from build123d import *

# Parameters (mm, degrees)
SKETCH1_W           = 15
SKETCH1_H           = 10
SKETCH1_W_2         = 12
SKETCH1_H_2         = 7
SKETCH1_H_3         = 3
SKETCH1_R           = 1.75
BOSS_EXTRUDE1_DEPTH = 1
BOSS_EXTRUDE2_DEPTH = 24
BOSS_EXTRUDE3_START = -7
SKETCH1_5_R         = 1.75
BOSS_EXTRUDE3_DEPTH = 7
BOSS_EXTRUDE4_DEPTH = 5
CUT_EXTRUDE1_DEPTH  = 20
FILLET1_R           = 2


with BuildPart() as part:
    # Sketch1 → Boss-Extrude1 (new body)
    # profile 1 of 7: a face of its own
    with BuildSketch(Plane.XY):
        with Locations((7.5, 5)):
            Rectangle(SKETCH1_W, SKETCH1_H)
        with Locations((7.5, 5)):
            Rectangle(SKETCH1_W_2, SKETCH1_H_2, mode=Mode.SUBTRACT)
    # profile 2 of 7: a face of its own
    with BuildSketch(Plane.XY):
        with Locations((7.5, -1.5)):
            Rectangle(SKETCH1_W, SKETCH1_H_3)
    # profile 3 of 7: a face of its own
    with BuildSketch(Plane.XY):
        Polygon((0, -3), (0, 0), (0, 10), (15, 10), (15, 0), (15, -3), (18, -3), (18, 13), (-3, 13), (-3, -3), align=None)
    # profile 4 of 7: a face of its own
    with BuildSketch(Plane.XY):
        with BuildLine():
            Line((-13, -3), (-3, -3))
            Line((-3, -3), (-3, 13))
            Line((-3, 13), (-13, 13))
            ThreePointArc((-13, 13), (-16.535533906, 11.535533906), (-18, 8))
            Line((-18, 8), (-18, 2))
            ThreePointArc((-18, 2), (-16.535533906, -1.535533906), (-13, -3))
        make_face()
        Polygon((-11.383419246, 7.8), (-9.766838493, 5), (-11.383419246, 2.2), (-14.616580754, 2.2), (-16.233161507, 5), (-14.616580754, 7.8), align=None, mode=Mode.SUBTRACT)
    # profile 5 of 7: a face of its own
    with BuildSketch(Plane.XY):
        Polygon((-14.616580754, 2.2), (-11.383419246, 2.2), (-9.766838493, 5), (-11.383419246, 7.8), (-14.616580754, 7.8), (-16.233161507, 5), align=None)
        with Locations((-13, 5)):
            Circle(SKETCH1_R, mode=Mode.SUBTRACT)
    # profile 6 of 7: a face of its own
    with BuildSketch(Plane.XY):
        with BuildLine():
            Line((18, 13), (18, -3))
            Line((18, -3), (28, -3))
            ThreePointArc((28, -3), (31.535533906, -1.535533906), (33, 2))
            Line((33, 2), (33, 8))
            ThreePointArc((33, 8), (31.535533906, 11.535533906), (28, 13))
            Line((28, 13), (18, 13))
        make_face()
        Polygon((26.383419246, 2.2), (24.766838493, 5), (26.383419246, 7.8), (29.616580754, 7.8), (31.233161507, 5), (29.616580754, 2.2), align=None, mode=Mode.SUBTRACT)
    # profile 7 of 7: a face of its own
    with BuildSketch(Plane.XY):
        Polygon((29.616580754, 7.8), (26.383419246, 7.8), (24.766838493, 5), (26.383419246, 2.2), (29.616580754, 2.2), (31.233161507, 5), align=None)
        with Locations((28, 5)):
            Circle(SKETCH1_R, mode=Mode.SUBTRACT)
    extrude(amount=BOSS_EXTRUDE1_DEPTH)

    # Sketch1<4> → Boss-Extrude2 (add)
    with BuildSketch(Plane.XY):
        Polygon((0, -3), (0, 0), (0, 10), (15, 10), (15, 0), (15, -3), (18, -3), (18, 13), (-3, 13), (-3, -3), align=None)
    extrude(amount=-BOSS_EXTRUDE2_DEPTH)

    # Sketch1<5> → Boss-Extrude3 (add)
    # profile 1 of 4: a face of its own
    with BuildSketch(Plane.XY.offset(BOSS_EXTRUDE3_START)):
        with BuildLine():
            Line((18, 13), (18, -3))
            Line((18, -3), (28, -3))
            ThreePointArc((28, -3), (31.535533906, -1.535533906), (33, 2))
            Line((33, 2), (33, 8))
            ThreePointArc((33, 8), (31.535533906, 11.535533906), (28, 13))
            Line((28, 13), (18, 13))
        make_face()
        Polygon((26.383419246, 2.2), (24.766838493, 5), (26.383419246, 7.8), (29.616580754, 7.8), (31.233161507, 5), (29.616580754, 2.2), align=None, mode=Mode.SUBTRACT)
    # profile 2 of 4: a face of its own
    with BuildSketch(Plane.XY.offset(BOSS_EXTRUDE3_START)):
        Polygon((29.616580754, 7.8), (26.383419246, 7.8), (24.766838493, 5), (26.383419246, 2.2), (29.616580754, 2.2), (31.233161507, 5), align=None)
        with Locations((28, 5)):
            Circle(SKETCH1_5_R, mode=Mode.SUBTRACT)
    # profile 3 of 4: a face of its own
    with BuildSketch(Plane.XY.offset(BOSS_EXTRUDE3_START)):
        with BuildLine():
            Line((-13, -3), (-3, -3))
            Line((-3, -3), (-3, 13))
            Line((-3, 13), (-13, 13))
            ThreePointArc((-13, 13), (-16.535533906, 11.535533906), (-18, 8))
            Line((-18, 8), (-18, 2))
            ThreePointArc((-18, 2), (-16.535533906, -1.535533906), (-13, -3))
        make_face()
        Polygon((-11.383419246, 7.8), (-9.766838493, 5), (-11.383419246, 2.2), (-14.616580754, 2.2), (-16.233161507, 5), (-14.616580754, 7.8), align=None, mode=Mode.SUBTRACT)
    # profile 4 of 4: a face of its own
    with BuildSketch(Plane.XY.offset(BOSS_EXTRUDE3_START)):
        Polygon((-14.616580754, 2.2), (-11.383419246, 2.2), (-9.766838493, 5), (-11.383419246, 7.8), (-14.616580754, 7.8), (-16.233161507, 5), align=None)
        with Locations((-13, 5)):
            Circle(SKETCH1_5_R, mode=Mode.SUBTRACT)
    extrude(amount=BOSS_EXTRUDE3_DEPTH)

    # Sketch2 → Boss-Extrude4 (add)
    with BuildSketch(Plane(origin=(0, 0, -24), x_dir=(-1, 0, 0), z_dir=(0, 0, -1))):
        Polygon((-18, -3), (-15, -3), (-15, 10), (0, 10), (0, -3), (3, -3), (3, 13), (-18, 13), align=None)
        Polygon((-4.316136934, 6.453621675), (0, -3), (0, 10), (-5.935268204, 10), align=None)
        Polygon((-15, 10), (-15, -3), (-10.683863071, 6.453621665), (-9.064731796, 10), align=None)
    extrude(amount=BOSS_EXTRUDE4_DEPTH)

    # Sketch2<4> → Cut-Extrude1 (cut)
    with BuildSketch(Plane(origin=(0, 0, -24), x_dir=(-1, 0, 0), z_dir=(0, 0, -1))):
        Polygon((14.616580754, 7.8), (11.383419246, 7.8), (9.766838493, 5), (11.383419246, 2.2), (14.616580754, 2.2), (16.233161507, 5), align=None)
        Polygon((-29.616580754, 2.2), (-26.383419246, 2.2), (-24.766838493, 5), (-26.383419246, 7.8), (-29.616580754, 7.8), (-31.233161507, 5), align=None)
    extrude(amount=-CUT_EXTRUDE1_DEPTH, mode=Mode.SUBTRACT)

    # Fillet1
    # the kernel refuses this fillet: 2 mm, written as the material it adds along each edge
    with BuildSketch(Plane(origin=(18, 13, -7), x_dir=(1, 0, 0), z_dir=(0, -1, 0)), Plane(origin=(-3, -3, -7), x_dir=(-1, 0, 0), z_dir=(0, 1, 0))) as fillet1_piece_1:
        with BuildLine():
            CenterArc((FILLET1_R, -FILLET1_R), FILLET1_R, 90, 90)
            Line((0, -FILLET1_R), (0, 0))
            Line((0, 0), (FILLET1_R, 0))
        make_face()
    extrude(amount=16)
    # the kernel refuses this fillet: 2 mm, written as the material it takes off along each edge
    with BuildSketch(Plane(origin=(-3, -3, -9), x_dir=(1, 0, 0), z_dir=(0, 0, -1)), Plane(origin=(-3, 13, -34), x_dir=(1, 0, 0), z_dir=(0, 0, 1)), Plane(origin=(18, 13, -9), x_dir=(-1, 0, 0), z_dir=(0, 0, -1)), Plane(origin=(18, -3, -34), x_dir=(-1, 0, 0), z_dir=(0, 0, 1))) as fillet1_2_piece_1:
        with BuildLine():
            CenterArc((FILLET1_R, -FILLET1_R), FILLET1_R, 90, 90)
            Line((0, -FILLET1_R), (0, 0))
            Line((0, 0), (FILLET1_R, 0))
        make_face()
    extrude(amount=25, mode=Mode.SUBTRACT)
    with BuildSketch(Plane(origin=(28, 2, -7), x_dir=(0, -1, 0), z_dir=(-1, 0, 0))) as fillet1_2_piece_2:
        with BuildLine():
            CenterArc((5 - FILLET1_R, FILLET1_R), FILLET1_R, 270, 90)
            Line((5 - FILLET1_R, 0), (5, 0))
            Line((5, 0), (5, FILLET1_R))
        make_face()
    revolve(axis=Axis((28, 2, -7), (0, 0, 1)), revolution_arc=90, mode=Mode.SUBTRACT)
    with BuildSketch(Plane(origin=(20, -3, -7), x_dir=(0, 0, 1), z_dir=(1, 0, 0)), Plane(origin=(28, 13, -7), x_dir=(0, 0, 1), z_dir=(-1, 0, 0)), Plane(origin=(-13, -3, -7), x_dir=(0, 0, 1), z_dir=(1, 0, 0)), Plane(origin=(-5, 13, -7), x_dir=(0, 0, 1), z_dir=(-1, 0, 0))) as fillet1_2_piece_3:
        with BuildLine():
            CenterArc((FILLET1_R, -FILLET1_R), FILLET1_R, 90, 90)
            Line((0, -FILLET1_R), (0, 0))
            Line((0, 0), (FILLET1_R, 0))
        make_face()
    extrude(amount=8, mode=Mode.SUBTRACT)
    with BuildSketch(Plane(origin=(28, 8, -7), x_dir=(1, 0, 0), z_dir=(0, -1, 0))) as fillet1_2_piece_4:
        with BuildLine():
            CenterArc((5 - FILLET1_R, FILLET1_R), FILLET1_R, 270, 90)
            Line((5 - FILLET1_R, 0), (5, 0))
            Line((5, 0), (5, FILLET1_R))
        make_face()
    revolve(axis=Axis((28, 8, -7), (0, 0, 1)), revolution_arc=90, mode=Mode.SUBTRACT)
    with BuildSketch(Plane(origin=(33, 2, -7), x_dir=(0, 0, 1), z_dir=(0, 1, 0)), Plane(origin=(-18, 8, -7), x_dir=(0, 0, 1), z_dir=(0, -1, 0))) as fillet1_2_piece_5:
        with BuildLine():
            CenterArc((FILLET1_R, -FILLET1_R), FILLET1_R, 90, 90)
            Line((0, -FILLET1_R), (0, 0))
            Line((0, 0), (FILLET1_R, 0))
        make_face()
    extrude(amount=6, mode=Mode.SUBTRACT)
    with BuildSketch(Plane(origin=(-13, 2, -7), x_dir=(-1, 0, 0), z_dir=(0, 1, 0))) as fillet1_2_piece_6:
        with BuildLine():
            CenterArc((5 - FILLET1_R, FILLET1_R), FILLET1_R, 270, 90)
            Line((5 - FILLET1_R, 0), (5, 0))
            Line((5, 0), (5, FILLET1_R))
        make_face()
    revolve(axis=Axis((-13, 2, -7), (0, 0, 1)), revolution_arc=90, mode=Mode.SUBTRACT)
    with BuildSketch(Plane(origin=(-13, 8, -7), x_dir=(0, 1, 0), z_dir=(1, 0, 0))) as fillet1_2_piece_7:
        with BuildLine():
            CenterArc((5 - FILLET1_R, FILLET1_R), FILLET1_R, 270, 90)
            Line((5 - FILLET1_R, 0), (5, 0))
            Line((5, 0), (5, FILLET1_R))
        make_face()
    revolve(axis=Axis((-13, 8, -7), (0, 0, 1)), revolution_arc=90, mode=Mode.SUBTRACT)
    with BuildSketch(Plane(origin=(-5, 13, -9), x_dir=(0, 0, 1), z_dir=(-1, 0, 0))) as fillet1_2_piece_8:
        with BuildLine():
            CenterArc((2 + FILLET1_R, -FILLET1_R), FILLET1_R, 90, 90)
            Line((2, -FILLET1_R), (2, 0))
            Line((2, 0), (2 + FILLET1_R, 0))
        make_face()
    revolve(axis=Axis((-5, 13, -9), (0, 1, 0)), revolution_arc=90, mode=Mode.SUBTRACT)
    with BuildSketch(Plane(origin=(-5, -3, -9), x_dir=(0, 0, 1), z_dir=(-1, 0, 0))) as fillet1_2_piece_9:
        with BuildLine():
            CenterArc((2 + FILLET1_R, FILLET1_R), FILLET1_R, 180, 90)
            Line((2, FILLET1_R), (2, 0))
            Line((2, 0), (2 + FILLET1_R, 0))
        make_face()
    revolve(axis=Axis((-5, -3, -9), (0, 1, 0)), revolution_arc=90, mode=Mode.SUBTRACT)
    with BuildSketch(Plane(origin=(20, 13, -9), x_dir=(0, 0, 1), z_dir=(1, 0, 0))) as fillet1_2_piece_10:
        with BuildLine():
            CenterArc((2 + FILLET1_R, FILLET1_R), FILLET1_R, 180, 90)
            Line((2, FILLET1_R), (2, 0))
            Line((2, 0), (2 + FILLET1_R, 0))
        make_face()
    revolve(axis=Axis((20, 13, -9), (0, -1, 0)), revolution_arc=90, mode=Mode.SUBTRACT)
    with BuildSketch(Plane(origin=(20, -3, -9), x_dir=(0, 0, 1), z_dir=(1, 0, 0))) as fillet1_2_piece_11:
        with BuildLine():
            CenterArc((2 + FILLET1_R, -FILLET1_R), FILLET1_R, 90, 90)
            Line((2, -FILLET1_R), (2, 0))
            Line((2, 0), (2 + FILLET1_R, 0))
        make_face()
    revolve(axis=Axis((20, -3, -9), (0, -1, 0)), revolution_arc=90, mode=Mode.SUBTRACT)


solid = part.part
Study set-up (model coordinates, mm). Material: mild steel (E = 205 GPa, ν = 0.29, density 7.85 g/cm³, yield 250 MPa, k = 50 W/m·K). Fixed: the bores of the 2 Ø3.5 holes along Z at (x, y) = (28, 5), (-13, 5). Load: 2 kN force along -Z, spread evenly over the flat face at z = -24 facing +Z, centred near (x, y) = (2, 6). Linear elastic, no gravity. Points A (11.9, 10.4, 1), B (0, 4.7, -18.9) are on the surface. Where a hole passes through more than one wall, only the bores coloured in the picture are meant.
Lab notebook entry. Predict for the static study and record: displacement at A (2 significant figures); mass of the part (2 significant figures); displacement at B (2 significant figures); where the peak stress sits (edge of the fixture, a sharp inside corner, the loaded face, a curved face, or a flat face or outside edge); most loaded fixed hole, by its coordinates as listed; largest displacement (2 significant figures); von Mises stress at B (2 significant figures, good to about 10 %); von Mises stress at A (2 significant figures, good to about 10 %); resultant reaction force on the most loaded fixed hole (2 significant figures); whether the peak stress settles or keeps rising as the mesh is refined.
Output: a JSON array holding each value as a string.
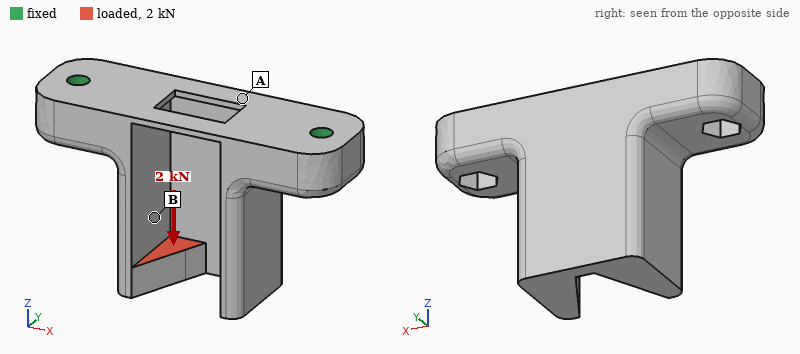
["6.4 µm", "63 g", "12 µm", "edge of the fixture", "(-13, 5)", "24 µm", "52 MPa", "20 MPa", "1.4 kN", "keeps rising"]
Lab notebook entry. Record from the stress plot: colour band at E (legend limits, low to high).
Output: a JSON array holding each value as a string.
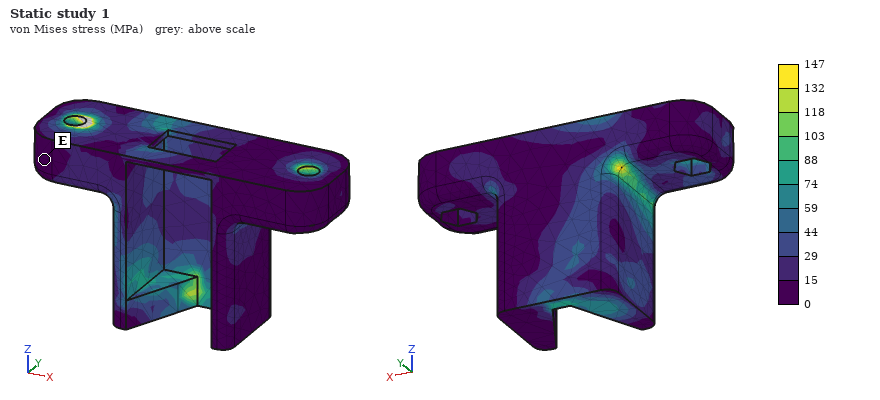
["0 to 15 MPa"]
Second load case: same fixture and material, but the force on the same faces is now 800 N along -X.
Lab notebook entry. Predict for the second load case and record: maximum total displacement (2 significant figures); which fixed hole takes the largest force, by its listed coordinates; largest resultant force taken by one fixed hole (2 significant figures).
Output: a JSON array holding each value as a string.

["44 µm", "(-13, 5)", "670 N"]
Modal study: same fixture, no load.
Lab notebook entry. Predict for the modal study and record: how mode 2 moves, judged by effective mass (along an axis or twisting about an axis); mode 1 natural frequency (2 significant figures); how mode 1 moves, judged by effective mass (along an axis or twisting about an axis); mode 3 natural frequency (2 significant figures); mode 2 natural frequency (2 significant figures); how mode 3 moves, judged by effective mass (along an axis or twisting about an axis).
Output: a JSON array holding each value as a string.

["along X", "5700 Hz", "along Y", "12 kHz", "7500 Hz", "along Z"]
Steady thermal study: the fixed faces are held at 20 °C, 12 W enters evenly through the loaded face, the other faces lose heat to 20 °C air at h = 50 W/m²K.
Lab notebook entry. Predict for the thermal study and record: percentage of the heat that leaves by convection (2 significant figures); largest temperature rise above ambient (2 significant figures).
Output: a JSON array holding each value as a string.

["32 %", "69 K"]
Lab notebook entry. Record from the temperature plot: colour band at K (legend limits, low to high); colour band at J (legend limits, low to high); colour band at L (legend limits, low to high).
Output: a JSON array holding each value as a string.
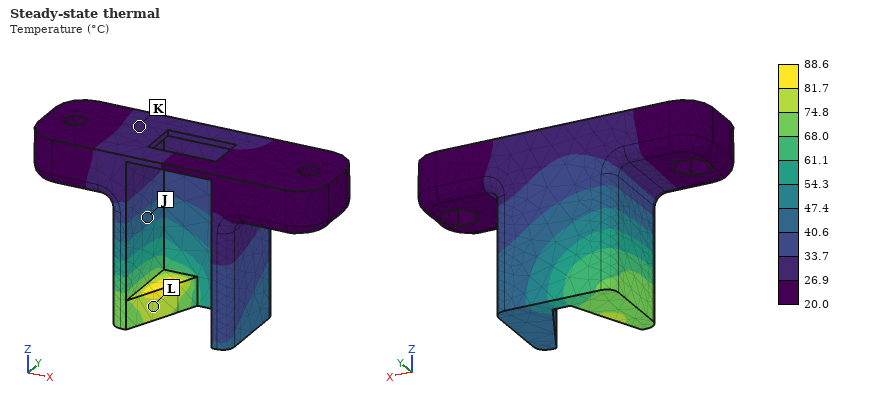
["26.9 to 33.7 °C", "40.6 to 47.4 °C", "74.8 to 81.7 °C"]
